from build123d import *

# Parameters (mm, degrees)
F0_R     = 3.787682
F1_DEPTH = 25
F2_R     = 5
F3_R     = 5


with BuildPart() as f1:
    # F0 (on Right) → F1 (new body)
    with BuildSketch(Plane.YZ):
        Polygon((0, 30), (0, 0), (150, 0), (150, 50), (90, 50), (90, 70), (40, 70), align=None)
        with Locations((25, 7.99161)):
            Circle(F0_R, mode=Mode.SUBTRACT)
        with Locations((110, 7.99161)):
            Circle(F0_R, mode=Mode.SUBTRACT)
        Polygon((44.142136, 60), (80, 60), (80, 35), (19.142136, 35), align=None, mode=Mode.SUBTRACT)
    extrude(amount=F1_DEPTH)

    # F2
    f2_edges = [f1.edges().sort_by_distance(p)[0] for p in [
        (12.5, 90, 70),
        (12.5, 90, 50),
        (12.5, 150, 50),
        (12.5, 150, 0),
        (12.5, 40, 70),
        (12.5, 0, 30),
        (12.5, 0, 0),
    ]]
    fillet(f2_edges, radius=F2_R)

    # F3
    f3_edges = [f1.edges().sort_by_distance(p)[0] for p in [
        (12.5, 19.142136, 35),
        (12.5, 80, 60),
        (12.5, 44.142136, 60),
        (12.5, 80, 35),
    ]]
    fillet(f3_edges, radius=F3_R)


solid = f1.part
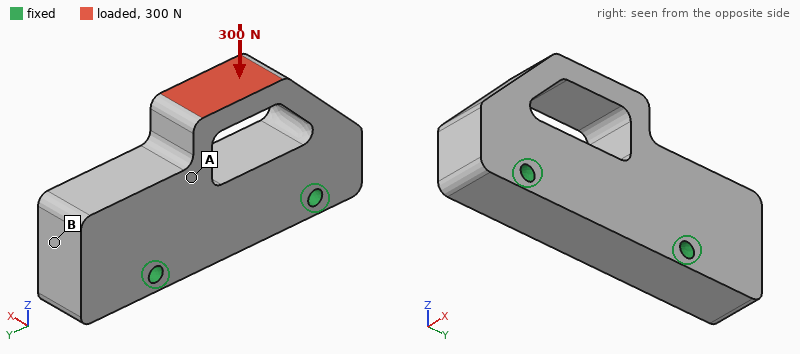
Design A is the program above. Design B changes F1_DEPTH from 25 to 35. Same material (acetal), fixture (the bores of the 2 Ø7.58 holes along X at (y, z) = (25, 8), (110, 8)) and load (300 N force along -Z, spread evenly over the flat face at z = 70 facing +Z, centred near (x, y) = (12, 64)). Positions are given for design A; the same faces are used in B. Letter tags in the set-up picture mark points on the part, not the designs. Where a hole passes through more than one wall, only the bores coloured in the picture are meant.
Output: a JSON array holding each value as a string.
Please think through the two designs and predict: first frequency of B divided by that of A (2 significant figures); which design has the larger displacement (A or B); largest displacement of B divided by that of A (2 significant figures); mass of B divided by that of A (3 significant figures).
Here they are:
["1.2", "A", "0.72", "1.40"]
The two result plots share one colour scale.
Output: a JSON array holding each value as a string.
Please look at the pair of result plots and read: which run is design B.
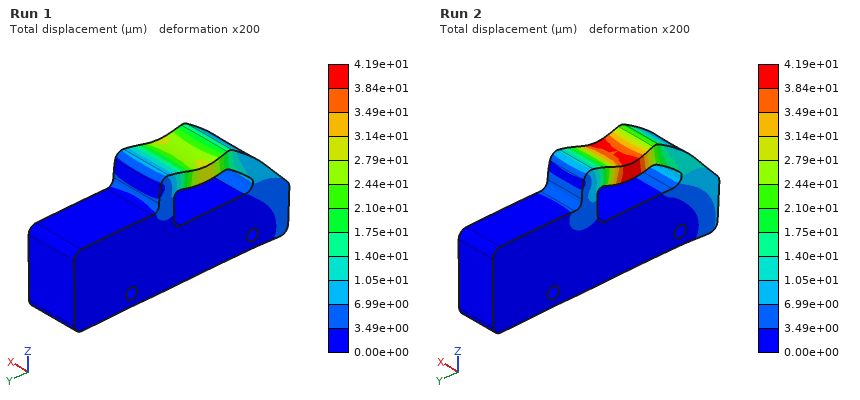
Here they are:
["Run 1"]
